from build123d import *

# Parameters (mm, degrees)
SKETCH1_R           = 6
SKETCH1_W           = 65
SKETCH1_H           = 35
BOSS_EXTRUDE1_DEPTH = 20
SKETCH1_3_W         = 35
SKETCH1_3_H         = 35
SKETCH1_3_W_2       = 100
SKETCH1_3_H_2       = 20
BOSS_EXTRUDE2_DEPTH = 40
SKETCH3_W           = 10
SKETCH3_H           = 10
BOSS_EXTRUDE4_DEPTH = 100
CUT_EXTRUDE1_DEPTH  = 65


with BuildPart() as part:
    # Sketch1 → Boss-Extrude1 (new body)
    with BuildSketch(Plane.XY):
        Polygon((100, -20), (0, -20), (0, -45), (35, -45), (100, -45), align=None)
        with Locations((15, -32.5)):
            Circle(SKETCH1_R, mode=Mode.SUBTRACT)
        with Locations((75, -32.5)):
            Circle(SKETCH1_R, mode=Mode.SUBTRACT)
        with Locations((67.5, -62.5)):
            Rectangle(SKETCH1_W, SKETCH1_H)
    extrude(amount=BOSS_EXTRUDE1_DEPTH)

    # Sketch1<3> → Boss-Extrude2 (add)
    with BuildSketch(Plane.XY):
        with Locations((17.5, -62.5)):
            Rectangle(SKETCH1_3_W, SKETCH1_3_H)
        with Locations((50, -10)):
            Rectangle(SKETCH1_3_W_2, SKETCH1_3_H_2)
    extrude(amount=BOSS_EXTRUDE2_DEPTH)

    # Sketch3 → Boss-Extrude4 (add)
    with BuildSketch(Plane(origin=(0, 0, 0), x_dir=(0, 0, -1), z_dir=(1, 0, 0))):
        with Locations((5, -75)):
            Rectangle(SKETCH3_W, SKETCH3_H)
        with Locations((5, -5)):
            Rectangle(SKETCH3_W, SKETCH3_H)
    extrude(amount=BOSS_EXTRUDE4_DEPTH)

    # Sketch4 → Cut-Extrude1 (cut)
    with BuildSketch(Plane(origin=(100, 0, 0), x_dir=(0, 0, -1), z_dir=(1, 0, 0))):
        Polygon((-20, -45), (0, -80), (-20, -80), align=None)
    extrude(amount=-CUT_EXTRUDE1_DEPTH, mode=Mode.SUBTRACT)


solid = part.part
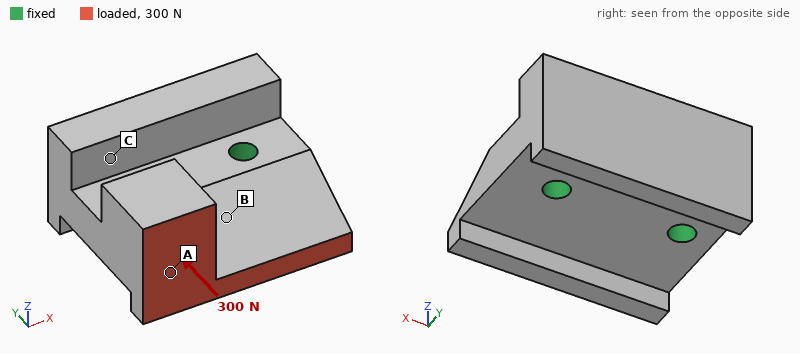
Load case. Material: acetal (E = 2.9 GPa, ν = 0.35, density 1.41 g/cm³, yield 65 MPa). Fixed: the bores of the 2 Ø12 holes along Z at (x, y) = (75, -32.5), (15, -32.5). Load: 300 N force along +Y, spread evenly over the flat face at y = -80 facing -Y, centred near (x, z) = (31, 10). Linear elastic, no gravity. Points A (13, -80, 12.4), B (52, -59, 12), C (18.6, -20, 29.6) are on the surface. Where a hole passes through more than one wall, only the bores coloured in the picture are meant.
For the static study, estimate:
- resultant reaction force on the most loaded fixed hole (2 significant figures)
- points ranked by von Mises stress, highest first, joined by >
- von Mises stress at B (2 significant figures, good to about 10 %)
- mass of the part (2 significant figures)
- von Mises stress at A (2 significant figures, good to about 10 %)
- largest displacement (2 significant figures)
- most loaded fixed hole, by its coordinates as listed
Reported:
220 N
A > B > C
0.21 MPa
310 g
0.31 MPa
43 µm
(15, -32.5)
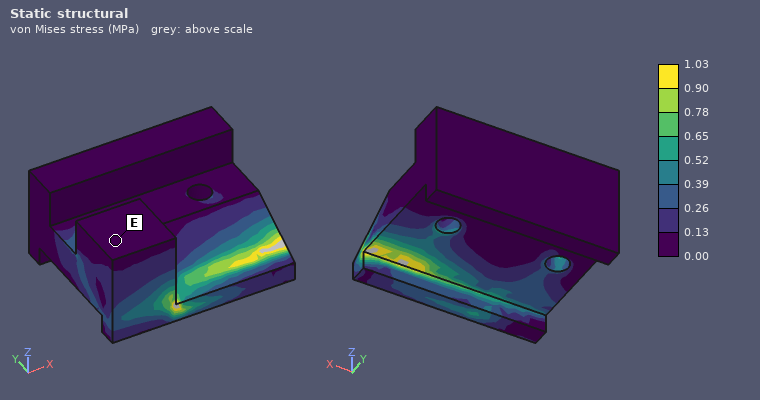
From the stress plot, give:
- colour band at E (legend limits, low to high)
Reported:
0.00 to 0.13 MPa
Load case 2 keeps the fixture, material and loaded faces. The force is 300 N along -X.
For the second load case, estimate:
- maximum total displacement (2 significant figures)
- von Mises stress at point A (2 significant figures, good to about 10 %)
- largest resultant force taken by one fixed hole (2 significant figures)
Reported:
33 µm
0.34 MPa
260 N
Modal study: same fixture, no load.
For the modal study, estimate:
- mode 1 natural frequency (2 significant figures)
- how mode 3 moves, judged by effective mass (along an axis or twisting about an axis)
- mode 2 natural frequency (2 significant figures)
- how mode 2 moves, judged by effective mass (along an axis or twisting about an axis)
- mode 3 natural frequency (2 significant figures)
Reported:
1300 Hz
along Z
1800 Hz
along Z
2000 Hz
